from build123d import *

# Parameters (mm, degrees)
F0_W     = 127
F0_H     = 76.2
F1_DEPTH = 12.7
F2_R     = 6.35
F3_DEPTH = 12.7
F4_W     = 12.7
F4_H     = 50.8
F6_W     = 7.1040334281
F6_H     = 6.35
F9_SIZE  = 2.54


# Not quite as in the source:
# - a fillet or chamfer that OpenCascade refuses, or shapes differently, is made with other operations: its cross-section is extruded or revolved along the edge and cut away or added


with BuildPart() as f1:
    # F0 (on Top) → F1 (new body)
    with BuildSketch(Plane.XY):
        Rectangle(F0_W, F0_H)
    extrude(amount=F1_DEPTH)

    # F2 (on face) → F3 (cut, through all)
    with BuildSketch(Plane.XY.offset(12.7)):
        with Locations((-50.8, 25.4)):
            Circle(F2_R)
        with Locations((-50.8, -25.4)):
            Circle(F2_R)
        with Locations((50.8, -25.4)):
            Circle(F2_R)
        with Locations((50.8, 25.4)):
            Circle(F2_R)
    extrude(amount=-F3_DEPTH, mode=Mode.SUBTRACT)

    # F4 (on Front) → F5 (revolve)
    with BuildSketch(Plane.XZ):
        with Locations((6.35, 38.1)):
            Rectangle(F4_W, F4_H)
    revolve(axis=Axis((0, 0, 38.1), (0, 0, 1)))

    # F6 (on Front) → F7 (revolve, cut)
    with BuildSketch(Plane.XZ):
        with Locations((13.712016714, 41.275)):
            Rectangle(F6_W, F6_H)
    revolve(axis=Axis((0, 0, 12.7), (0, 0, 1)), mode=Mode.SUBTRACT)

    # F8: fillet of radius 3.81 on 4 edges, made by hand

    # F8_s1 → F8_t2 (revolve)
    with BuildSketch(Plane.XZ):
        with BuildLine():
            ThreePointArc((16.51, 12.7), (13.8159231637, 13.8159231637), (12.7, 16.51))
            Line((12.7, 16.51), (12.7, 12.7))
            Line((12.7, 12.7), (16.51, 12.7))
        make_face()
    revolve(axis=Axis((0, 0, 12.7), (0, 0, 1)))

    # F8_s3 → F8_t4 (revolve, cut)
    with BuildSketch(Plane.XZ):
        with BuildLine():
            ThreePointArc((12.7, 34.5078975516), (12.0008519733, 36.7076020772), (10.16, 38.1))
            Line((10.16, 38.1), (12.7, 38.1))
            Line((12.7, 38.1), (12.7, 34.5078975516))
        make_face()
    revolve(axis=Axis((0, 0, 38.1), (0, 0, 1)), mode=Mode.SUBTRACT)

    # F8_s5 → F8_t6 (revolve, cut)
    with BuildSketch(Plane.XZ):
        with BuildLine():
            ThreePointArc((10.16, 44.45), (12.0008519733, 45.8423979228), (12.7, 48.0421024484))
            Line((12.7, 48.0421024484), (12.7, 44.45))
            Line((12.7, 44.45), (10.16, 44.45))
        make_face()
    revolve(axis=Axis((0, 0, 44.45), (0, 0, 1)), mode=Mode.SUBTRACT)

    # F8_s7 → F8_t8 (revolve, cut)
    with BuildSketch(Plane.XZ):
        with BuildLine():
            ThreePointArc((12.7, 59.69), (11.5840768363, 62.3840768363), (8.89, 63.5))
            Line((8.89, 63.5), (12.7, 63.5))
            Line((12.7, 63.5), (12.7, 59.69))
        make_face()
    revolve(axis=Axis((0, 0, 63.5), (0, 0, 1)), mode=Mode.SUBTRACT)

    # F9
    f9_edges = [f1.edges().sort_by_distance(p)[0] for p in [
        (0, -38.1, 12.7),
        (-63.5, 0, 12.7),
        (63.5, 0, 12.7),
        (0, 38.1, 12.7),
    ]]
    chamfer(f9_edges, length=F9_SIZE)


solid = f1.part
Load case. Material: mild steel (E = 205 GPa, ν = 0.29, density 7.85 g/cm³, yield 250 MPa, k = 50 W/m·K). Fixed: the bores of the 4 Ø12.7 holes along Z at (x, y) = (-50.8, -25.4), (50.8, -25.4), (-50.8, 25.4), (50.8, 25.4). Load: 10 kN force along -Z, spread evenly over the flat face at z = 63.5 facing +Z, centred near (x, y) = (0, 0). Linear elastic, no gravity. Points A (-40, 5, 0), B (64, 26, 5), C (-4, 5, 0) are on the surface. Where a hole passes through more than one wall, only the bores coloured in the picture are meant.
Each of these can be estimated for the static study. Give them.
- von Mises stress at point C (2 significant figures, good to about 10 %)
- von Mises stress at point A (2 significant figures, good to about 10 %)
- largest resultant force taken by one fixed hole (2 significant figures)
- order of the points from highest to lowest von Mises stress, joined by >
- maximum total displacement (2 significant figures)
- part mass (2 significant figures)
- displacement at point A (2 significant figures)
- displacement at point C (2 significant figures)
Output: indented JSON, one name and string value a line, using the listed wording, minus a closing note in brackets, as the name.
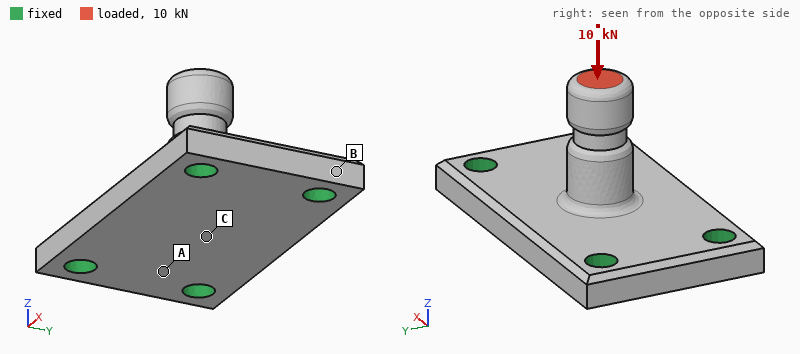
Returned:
{
  "von Mises stress at point C": "37 MPa",
  "von Mises stress at point A": "20 MPa",
  "largest resultant force taken by one fixed hole": "2.5 kN",
  "order of the points from highest to lowest von Mises stress, joined by >": "C > A > B",
  "maximum total displacement": "25 µm",
  "part mass": "1.1 kg",
  "displacement at point A": "4.8 µm",
  "displacement at point C": "19 µm"
}
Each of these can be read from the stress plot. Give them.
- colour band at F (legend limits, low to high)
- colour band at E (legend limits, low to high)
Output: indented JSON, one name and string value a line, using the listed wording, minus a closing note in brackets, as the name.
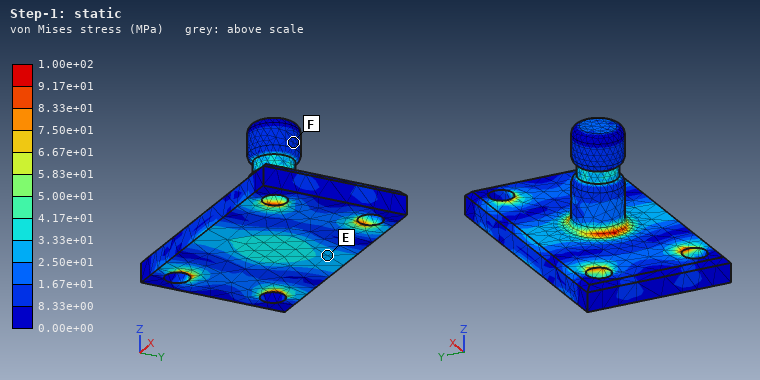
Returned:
{
  "colour band at F": "8.33e+00 to 1.67e+01 MPa",
  "colour band at E": "2.50e+01 to 3.33e+01 MPa"
}
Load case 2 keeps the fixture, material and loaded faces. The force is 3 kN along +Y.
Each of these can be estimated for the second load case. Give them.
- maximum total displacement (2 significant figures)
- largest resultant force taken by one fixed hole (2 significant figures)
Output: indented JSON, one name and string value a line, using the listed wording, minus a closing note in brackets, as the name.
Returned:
{
  "maximum total displacement": "79 µm",
  "largest resultant force taken by one fixed hole": "1.9 kN"
}
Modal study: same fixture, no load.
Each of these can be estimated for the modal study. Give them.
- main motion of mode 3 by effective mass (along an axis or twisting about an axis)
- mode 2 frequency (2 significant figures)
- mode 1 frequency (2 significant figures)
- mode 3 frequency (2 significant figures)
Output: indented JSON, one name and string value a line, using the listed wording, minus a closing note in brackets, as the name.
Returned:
{
  "main motion of mode 3 by effective mass": "along Z",
  "mode 2 frequency": "4600 Hz",
  "mode 1 frequency": "3900 Hz",
  "mode 3 frequency": "5200 Hz"
}
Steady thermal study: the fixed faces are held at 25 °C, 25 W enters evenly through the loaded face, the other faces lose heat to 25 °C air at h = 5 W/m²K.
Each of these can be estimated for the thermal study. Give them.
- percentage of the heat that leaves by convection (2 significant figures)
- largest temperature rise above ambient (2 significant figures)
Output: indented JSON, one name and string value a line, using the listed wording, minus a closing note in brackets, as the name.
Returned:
{
  "percentage of the heat that leaves by convection": "5.5 %",
  "largest temperature rise above ambient": "74 K"
}
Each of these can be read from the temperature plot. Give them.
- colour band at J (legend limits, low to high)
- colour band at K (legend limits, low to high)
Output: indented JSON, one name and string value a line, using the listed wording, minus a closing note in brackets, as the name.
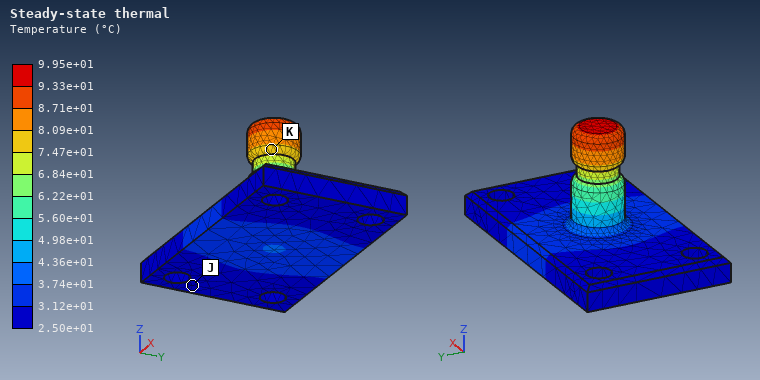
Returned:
{
  "colour band at J": "2.50e+01 to 3.12e+01 °C",
  "colour band at K": "7.47e+01 to 8.09e+01 °C"
}
